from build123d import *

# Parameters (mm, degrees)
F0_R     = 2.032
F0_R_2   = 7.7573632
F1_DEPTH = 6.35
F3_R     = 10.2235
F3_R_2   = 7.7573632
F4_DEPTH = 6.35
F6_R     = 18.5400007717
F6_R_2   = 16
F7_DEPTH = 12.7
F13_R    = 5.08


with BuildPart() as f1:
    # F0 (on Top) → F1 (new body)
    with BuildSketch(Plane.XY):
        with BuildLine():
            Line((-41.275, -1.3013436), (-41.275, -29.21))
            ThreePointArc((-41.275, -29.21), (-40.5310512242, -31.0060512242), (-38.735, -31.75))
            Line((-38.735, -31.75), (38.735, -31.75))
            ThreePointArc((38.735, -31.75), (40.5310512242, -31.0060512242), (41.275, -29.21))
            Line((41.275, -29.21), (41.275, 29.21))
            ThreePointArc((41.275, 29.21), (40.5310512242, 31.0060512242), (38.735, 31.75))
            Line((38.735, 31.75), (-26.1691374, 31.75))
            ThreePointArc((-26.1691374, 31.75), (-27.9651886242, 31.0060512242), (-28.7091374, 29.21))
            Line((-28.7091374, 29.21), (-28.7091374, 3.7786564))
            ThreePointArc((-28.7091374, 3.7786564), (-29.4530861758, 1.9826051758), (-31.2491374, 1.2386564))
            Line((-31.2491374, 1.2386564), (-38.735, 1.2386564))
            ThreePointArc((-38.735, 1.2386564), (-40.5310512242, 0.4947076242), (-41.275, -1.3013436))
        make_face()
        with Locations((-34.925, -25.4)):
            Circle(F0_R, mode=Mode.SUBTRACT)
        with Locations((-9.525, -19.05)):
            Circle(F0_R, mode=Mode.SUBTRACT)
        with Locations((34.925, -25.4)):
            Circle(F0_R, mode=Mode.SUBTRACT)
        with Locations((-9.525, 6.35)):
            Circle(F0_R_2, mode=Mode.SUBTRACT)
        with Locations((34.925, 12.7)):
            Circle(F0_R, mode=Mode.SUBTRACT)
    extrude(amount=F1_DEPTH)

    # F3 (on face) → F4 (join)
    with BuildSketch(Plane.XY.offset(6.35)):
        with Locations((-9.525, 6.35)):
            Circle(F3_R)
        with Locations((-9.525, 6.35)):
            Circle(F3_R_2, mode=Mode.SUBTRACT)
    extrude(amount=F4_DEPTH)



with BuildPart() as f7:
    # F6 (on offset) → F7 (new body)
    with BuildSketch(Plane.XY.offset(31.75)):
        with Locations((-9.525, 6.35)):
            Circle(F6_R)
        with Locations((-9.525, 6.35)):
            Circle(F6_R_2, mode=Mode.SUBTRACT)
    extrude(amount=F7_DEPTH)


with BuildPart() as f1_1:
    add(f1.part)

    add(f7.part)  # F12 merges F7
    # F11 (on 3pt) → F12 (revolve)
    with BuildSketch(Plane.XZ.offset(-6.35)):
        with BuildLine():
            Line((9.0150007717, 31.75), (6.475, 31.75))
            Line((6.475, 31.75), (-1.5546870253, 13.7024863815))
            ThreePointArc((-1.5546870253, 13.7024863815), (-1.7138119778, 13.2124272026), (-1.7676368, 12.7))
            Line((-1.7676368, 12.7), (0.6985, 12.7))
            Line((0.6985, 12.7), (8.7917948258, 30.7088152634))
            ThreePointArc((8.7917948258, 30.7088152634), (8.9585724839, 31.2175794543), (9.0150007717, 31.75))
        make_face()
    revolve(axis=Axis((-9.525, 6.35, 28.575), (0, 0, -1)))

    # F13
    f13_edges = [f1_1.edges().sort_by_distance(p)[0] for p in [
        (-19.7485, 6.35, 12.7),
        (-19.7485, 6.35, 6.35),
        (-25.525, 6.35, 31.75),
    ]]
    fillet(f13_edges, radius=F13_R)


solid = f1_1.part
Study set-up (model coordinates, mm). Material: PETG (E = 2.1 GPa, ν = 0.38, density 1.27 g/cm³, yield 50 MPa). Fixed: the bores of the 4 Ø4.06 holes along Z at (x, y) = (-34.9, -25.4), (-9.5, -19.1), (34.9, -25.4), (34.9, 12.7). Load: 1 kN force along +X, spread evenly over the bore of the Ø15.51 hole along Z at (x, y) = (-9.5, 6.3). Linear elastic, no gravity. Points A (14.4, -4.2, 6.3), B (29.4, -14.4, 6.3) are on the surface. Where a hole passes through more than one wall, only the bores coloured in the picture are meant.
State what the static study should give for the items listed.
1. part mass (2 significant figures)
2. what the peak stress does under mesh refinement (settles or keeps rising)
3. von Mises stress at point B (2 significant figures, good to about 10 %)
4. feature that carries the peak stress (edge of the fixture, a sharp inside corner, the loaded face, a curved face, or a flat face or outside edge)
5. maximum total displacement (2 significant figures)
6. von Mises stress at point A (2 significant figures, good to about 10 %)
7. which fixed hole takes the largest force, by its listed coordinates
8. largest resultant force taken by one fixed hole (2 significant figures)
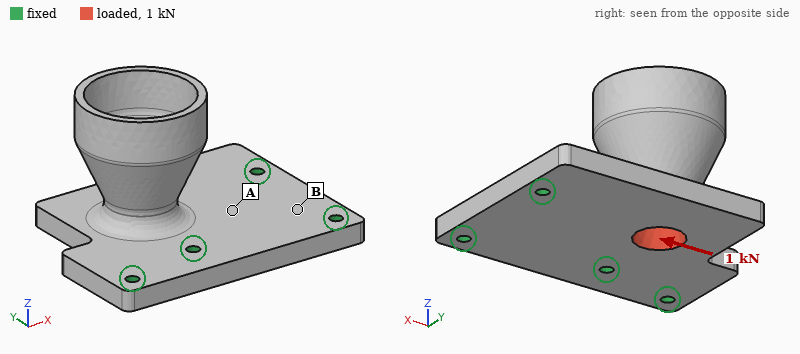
49 g
keeps rising
1.5 MPa
edge of the fixture
0.48 mm
3.2 MPa
(34.9, 12.7)
430 N
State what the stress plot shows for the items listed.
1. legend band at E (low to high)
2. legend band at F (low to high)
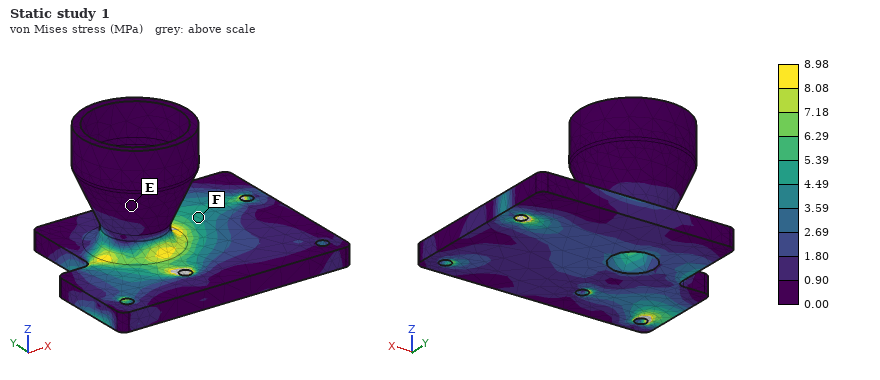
0.00 to 0.90 MPa
4.49 to 5.39 MPa
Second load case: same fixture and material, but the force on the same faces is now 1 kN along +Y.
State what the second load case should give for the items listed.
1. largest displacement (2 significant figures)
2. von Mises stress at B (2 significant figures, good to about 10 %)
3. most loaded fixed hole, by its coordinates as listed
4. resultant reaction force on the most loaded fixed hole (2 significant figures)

0.81 mm
2.6 MPa
(-9.5, -19.1)
570 N
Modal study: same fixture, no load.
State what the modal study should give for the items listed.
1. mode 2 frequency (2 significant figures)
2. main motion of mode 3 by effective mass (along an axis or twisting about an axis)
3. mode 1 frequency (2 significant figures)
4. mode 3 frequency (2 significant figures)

870 Hz
along Z
480 Hz
1500 Hz
